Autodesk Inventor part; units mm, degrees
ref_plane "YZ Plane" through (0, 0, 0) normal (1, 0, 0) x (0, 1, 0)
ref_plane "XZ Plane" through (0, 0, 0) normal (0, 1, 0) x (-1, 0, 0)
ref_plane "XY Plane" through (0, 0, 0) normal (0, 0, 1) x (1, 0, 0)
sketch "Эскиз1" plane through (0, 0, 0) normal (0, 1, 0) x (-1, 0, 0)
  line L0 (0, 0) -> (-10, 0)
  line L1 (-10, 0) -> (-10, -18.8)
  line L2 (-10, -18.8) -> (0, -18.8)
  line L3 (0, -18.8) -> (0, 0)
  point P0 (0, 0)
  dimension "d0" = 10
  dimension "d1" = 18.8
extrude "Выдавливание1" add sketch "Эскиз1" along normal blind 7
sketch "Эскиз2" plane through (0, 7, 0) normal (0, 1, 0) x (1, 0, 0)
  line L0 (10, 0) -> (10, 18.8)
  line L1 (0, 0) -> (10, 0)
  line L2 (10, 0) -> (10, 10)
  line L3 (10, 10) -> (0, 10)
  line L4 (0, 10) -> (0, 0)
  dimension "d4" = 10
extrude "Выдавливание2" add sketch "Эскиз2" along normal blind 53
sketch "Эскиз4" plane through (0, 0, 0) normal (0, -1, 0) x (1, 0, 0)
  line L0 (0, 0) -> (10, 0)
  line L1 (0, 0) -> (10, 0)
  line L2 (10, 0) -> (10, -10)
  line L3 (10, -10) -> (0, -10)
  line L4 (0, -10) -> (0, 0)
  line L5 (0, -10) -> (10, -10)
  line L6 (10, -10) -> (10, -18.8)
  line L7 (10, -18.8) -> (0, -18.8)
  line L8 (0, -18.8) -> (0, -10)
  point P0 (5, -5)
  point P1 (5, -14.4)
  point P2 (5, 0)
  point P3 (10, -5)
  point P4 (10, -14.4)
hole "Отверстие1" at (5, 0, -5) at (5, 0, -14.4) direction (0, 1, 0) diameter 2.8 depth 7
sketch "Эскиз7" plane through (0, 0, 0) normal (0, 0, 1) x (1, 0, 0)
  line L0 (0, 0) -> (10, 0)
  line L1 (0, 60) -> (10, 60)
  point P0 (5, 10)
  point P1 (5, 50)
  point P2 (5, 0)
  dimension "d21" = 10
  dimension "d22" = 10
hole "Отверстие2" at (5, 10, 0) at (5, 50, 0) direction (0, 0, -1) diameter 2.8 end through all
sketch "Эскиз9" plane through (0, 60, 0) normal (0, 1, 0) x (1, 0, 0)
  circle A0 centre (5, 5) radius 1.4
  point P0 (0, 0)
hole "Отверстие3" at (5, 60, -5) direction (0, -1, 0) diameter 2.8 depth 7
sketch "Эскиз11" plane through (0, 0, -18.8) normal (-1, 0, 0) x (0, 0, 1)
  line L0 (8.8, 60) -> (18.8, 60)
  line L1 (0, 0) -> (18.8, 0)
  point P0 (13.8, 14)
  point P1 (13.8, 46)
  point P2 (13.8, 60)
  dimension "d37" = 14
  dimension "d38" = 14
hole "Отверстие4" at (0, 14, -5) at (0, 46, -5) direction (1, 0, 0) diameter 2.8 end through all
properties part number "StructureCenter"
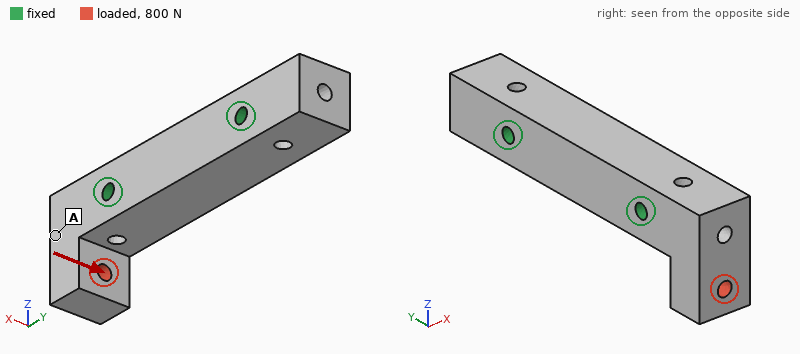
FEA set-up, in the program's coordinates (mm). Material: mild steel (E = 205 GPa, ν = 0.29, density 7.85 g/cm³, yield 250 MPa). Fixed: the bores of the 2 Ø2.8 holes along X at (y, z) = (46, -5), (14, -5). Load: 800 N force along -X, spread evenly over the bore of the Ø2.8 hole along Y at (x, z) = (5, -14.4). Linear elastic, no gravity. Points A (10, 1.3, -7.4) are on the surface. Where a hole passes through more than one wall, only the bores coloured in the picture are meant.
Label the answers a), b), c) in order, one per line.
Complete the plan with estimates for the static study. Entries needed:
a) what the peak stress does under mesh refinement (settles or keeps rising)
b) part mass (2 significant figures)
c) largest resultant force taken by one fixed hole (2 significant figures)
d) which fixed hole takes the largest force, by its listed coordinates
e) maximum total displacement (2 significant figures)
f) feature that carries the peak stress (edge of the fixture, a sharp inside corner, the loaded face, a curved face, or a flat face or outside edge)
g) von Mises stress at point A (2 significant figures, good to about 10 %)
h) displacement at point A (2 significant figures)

a) keeps rising
b) 49 g
c) 830 N
d) (14, -5)
e) 17 µm
f) edge of the fixture
g) 23 MPa
h) 6.8 µm
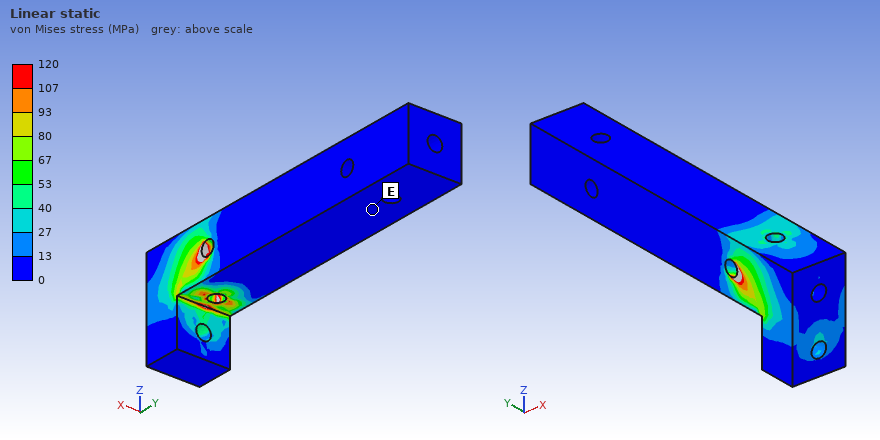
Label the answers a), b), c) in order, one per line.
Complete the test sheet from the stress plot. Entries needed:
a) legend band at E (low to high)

a) 0 to 13 MPa
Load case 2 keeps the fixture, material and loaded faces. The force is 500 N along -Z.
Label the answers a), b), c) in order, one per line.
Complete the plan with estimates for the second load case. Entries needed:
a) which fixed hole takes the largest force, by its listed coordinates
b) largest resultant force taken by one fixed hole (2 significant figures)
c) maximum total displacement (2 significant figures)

a) (14, -5)
b) 580 N
c) 7.2 µm
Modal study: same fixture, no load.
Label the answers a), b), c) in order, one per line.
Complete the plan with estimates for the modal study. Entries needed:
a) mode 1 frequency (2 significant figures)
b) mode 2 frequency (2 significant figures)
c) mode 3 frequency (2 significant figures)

a) 14 kHz
b) 17 kHz
c) 23 kHz
